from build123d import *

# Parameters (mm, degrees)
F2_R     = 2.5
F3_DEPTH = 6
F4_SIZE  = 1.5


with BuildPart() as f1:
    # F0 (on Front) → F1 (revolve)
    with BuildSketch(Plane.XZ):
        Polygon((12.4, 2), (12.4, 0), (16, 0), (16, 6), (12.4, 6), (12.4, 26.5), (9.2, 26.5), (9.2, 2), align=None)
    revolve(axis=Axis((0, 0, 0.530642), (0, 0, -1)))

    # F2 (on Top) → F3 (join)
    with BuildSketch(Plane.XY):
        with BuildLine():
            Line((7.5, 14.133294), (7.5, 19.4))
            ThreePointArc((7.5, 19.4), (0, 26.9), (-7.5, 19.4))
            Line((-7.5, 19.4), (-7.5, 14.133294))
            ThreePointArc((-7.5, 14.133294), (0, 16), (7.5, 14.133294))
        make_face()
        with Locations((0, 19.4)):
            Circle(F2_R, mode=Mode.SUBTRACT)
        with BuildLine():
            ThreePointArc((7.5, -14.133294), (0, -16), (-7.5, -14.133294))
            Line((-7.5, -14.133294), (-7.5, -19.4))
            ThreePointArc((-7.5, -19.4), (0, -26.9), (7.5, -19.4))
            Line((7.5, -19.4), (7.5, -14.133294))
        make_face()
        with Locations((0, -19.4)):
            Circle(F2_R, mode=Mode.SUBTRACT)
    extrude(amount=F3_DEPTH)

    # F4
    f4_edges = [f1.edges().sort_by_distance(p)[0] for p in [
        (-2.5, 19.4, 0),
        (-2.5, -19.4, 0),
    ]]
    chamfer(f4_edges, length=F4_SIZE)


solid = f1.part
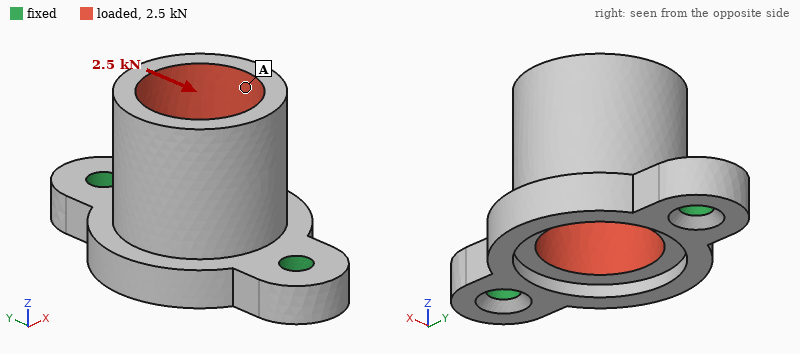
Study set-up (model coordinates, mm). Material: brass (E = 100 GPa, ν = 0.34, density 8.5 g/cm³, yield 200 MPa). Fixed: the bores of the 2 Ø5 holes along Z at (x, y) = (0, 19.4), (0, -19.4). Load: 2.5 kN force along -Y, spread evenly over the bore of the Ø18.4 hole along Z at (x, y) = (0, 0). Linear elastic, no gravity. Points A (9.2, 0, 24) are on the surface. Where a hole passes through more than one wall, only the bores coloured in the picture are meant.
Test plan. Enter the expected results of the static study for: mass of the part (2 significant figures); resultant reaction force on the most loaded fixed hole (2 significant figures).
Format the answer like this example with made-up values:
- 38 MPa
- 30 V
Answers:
- 74 g
- 1.5 kN
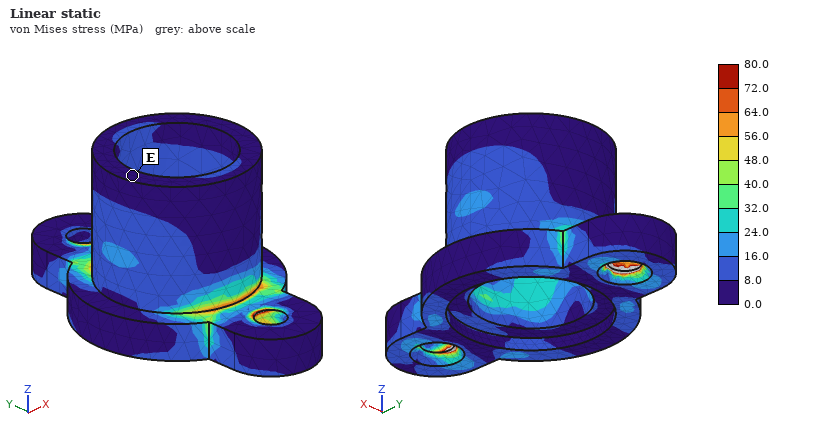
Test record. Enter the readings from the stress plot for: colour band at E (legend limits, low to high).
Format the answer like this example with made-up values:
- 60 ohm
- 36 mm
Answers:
- 0.0 to 8.0 MPa
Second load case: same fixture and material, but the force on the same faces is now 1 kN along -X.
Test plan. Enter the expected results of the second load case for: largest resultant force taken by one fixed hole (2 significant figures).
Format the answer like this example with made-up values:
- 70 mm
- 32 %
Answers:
- 500 N
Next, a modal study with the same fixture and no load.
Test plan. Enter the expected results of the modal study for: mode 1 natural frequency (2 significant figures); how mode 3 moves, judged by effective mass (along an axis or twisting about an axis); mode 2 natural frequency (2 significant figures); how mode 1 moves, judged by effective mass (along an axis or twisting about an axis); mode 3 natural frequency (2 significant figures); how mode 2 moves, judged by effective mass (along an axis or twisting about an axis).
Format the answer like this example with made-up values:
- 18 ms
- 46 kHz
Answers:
- 3600 Hz
- along Y
- 8600 Hz
- along X
- 9400 Hz
- along Z
